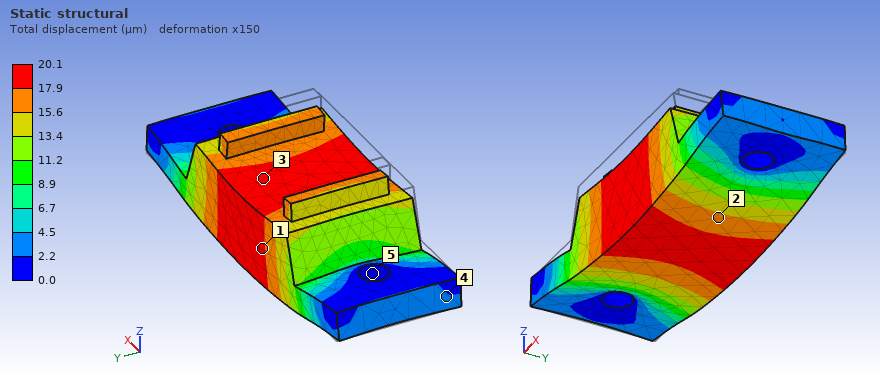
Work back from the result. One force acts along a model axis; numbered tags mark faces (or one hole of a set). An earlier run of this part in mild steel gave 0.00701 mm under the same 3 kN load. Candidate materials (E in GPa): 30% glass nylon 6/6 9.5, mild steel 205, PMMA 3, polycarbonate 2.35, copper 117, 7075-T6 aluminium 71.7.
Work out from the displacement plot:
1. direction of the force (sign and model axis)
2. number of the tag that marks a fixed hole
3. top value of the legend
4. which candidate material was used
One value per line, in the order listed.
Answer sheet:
-Z
5
20.1 µm
7075-T6 aluminium
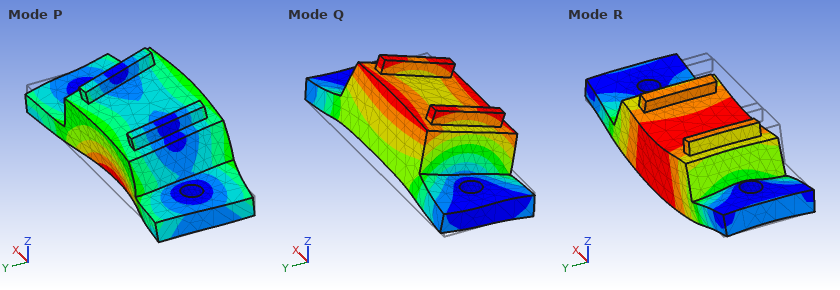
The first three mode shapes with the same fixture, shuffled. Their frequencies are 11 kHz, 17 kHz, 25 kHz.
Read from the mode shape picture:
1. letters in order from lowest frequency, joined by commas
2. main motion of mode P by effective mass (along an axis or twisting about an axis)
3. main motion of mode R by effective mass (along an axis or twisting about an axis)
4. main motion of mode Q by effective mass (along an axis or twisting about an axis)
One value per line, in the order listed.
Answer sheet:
Q, R, P
along Y
along Z
along Y
